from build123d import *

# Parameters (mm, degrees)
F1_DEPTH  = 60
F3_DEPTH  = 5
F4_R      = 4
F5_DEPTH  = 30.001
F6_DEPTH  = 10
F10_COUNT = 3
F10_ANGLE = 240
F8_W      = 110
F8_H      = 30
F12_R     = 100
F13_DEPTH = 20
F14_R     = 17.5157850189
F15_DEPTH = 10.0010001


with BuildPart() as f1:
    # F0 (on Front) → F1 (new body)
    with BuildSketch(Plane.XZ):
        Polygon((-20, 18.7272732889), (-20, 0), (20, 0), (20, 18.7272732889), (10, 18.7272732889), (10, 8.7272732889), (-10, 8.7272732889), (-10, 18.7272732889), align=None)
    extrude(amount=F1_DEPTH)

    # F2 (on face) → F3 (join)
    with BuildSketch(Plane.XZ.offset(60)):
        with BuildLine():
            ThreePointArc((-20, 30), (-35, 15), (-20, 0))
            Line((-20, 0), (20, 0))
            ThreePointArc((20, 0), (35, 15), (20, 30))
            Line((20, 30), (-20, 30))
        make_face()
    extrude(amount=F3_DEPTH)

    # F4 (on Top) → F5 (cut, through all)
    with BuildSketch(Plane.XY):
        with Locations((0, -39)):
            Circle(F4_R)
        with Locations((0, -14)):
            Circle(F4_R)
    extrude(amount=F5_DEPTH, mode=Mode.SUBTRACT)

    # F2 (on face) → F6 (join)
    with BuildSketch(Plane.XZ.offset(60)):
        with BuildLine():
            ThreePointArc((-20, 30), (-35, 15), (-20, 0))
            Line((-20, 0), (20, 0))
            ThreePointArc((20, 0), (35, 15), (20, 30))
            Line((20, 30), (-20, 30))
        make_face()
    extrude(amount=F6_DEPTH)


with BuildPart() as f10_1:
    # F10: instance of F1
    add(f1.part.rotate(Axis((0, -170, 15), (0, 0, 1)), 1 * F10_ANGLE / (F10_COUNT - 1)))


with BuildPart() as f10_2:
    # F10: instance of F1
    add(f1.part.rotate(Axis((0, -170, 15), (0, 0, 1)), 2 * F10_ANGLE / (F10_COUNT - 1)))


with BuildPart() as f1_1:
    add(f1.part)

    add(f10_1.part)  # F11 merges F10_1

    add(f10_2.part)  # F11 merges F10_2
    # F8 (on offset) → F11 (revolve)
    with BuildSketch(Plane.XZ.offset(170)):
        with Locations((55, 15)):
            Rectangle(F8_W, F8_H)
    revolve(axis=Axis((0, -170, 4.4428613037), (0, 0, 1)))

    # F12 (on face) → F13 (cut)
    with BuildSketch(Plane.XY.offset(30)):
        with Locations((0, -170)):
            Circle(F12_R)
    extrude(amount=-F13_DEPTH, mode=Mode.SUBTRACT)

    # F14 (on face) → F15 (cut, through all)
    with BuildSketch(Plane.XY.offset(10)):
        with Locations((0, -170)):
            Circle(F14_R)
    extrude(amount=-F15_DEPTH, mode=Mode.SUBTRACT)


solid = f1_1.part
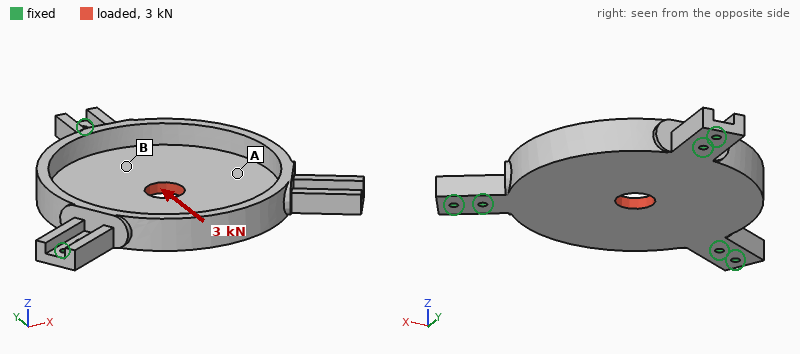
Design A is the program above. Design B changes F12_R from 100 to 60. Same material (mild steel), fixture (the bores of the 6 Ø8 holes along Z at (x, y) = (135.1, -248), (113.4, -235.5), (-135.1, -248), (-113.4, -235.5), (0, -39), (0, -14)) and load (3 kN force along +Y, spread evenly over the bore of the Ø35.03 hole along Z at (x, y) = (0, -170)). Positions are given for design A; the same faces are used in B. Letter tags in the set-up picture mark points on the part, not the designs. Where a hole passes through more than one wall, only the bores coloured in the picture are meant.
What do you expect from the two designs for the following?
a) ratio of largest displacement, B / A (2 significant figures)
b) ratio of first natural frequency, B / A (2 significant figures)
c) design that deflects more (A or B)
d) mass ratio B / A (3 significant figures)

0.83
1.2
A
1.66
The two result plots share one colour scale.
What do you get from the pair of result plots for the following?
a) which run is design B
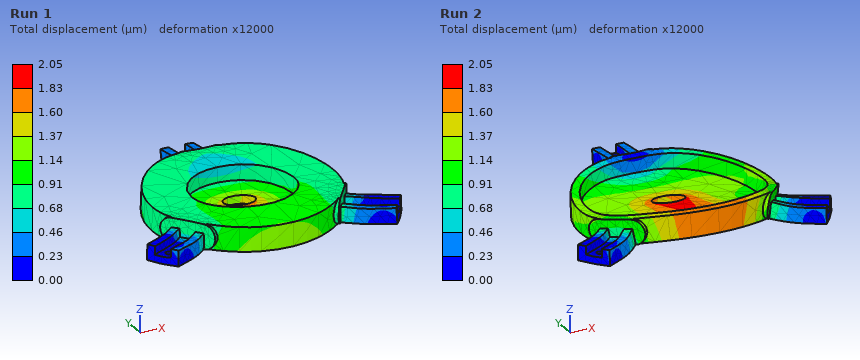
Run 1
